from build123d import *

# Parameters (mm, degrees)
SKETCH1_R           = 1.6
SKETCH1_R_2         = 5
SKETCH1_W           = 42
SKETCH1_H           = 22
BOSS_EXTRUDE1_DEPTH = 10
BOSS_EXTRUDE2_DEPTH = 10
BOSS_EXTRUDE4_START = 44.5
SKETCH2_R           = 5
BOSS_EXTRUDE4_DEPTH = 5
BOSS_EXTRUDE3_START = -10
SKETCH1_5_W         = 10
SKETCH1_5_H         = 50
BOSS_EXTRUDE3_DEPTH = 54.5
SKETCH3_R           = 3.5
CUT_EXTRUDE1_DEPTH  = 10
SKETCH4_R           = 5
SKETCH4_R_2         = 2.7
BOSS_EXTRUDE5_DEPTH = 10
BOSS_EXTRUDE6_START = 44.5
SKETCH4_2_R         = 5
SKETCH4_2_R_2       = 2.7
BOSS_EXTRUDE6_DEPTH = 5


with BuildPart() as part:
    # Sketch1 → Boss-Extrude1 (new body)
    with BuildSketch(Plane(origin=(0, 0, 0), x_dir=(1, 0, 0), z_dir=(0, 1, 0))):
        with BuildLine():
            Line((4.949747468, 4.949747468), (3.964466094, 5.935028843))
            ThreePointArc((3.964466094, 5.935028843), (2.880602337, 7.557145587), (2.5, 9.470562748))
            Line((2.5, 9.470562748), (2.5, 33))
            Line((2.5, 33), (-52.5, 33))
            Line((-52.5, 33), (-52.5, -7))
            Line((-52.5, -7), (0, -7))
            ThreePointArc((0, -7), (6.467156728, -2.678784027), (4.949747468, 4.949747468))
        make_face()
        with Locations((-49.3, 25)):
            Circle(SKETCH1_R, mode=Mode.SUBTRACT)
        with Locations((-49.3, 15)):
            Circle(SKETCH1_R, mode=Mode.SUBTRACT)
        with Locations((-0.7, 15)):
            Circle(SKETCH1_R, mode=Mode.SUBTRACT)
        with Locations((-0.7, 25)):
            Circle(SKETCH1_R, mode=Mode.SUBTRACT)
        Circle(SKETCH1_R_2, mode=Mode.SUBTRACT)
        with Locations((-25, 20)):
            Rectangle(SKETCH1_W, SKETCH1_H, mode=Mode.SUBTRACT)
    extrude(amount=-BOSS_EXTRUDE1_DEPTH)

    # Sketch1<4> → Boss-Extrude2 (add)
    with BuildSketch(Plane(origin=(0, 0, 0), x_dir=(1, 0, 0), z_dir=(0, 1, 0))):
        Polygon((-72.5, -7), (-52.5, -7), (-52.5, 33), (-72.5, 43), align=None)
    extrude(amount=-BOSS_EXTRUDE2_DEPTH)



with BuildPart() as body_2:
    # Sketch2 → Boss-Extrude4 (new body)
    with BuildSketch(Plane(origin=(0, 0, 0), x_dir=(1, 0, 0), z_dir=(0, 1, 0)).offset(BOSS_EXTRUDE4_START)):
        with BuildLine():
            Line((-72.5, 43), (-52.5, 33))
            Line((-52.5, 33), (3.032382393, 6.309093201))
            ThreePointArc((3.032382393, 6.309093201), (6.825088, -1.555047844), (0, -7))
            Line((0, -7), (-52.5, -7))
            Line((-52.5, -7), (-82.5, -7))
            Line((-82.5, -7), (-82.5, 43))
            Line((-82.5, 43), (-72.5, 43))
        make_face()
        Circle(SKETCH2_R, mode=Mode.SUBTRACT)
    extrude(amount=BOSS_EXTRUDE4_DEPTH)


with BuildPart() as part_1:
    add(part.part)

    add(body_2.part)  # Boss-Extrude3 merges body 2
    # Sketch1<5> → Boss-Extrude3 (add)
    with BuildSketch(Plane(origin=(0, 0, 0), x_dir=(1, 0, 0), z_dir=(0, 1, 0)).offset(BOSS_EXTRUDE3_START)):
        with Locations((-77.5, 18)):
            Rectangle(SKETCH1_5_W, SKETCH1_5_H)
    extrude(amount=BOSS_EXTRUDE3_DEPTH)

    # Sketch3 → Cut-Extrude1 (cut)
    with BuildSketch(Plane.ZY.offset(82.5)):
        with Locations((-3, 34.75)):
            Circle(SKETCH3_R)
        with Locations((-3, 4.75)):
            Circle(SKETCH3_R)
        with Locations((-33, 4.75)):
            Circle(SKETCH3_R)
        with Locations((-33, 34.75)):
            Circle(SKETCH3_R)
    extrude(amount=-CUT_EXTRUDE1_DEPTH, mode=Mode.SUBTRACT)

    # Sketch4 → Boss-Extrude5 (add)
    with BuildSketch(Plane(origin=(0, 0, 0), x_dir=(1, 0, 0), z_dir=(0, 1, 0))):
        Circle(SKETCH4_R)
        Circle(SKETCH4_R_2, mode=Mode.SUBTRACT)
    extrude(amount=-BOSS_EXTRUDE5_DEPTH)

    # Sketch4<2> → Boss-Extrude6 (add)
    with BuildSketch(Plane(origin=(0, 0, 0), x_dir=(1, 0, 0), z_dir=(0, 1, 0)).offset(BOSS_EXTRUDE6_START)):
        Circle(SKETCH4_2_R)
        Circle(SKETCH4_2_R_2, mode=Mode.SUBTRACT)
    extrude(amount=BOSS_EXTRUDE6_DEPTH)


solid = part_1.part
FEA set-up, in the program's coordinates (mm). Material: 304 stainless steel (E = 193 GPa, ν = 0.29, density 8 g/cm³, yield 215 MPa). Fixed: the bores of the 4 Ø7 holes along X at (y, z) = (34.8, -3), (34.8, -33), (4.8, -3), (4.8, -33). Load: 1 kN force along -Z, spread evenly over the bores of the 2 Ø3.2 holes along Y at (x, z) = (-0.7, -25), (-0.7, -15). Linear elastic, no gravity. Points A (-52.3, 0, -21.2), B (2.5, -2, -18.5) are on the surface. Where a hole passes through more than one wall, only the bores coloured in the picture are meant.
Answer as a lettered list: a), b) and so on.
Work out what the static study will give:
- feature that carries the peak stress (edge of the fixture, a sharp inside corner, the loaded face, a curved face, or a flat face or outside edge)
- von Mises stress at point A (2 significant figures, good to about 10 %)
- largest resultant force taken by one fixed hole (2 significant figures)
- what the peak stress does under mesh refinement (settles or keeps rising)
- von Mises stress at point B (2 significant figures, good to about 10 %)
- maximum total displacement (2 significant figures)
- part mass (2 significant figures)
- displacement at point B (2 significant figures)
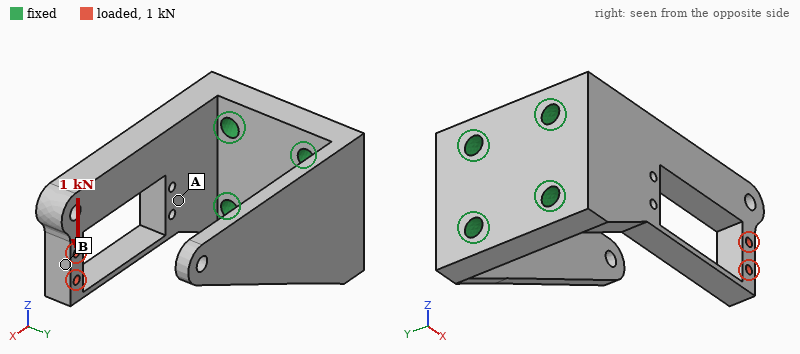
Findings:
a) edge of the fixture
b) 15 MPa
c) 2.3 kN
d) keeps rising
e) 38 MPa
f) 91 µm
g) 490 g
h) 80 µm
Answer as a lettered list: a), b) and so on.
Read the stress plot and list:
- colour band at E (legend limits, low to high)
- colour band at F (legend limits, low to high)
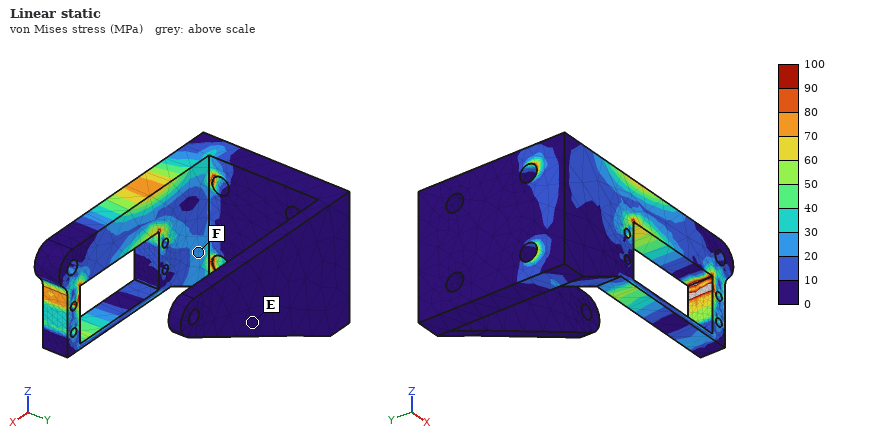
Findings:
a) 0 to 10 MPa
b) 20 to 30 MPa
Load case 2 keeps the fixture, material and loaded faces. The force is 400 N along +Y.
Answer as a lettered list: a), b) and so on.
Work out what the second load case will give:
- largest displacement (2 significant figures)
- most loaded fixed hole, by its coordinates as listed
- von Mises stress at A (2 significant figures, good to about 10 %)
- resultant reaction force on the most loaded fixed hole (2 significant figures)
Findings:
a) 0.18 mm
b) (4.8, -33)
c) 14 MPa
d) 260 N
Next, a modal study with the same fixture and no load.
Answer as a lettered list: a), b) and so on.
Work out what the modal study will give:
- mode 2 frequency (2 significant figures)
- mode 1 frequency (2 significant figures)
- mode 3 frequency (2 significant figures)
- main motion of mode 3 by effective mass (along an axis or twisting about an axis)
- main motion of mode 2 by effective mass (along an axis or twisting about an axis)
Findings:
a) 1300 Hz
b) 870 Hz
c) 2800 Hz
d) along Z
e) along Y
